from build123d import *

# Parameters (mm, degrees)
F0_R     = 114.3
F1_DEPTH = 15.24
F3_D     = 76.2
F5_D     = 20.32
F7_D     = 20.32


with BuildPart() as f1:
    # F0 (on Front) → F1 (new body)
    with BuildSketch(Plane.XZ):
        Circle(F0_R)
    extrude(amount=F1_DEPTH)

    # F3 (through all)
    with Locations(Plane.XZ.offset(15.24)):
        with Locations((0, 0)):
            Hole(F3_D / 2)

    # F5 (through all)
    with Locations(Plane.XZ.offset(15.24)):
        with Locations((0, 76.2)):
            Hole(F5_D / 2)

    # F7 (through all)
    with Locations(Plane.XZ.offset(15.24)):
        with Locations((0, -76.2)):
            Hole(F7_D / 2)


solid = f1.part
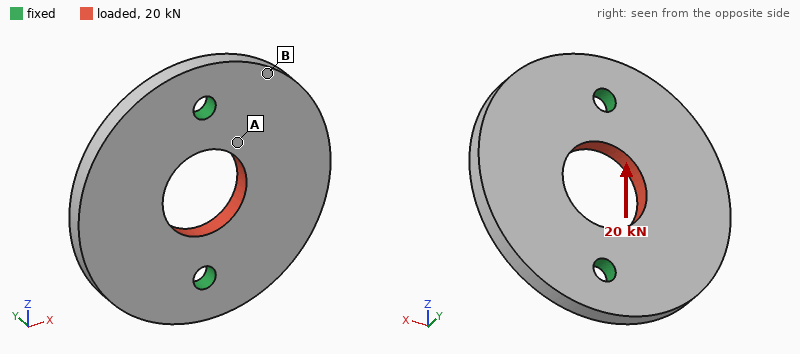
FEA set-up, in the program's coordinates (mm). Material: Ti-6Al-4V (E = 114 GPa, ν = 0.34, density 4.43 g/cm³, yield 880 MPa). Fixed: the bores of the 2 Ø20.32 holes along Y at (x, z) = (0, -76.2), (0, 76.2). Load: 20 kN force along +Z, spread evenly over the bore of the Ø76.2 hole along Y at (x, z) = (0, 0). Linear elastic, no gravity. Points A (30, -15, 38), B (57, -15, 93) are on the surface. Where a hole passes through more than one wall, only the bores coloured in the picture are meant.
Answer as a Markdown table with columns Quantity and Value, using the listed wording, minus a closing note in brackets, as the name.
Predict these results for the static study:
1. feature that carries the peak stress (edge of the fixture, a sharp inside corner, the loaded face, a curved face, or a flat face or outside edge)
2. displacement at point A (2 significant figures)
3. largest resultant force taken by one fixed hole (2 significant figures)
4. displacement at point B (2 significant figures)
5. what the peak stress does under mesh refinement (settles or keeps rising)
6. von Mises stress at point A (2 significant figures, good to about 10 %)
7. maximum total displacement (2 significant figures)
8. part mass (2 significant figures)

| Quantity | Value |
|---|---|
| feature that carries the peak stress | edge of the fixture |
| displacement at point A | 4.5 µm |
| largest resultant force taken by one fixed hole | 10 kN |
| displacement at point B | 3.8 µm |
| what the peak stress does under mesh refinement | keeps rising |
| von Mises stress at point A | 7.9 MPa |
| maximum total displacement | 6.5 µm |
| part mass | 2.4 kg |
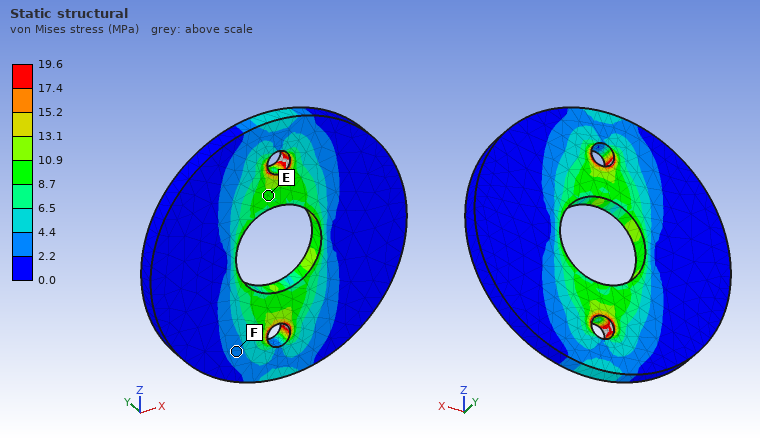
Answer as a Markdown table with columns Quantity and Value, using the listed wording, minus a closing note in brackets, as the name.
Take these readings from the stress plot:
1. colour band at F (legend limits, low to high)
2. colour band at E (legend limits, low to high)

| Quantity | Value |
|---|---|
| colour band at F | 2.2 to 4.4 MPa |
| colour band at E | 8.7 to 10.9 MPa |
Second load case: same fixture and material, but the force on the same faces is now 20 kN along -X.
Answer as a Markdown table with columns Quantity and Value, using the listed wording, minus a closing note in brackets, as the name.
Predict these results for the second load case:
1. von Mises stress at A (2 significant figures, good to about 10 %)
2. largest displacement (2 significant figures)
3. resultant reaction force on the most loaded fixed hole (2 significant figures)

| Quantity | Value |
|---|---|
| von Mises stress at A | 7.1 MPa |
| largest displacement | 7.3 µm |
| resultant reaction force on the most loaded fixed hole | 10 kN |
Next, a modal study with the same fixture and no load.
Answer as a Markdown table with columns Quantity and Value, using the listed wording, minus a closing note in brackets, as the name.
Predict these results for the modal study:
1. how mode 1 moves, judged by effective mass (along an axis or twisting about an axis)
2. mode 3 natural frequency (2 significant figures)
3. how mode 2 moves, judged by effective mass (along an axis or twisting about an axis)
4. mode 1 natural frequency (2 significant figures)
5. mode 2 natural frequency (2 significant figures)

| Quantity | Value |
|---|---|
| how mode 1 moves, judged by effective mass | twisting about Z |
| mode 3 natural frequency | 2500 Hz |
| how mode 2 moves, judged by effective mass | along Y |
| mode 1 natural frequency | 1000 Hz |
| mode 2 natural frequency | 1100 Hz |
